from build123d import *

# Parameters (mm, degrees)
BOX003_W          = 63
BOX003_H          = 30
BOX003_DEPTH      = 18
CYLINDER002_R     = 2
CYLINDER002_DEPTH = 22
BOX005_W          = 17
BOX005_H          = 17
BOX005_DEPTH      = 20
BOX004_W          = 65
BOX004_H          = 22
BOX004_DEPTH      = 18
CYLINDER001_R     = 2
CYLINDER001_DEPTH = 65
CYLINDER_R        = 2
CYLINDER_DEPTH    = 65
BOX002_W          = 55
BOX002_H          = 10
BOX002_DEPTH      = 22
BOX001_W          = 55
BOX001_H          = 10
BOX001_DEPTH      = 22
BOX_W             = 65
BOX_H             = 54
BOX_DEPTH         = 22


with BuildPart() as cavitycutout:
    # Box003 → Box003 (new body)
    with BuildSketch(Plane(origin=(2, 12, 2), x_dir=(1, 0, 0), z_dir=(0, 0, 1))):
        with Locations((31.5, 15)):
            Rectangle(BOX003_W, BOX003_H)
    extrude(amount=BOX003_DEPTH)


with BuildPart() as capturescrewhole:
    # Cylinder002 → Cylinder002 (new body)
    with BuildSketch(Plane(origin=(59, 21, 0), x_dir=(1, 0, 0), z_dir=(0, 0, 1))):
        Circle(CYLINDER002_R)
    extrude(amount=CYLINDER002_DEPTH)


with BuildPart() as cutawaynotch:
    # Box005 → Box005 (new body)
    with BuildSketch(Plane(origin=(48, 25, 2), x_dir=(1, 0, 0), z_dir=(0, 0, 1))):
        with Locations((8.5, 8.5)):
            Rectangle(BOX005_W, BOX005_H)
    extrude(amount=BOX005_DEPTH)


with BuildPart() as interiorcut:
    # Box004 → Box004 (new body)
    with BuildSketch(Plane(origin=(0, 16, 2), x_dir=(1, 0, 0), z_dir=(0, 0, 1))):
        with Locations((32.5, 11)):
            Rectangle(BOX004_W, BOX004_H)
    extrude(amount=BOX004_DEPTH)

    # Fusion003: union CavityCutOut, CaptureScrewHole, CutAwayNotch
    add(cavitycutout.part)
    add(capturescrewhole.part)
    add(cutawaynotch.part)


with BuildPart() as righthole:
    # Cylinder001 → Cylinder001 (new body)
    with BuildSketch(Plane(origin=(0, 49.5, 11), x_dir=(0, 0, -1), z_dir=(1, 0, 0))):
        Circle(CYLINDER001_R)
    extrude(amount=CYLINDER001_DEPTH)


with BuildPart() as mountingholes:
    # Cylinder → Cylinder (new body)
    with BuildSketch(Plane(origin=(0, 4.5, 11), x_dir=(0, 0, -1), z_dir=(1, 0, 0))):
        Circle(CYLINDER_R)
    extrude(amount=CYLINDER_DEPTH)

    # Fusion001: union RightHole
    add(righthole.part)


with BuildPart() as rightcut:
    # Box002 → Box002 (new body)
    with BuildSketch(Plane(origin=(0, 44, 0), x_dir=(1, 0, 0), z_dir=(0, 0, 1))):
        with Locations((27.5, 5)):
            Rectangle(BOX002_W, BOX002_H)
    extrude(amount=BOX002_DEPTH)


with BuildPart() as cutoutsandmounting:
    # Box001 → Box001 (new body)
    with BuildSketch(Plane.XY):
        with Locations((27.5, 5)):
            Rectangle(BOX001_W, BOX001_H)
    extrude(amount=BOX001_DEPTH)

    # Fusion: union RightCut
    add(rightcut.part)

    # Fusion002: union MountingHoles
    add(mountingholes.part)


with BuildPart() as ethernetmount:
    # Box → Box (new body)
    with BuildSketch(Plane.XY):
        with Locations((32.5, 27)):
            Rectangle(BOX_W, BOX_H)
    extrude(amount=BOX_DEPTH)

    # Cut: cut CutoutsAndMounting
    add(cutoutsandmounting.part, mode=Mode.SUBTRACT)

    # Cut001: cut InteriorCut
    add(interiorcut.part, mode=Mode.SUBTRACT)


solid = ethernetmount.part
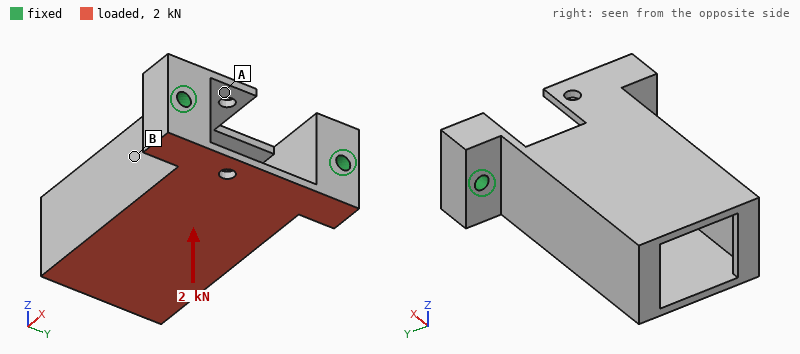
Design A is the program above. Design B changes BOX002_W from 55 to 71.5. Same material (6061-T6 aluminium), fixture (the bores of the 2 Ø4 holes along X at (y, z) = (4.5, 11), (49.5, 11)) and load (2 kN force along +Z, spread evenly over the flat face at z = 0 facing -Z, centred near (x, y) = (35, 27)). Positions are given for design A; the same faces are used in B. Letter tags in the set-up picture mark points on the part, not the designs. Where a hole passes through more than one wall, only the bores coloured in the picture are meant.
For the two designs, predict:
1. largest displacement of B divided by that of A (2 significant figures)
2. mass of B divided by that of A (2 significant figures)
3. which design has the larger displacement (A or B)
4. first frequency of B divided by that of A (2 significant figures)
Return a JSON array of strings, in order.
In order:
["2.4", "0.90", "B", "0.66"]
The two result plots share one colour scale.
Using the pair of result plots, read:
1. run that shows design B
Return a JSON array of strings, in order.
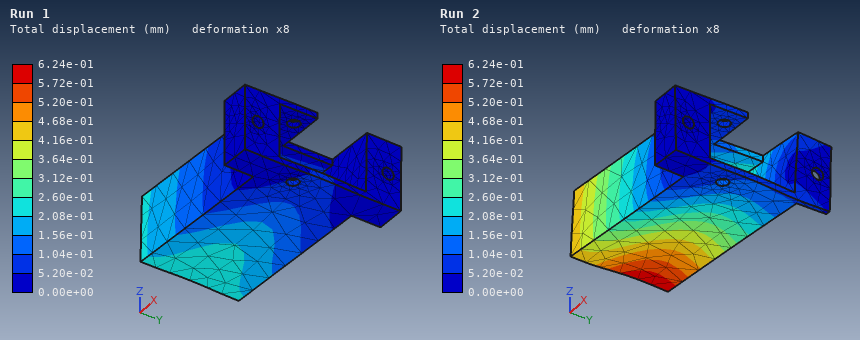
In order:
["Run 2"]
